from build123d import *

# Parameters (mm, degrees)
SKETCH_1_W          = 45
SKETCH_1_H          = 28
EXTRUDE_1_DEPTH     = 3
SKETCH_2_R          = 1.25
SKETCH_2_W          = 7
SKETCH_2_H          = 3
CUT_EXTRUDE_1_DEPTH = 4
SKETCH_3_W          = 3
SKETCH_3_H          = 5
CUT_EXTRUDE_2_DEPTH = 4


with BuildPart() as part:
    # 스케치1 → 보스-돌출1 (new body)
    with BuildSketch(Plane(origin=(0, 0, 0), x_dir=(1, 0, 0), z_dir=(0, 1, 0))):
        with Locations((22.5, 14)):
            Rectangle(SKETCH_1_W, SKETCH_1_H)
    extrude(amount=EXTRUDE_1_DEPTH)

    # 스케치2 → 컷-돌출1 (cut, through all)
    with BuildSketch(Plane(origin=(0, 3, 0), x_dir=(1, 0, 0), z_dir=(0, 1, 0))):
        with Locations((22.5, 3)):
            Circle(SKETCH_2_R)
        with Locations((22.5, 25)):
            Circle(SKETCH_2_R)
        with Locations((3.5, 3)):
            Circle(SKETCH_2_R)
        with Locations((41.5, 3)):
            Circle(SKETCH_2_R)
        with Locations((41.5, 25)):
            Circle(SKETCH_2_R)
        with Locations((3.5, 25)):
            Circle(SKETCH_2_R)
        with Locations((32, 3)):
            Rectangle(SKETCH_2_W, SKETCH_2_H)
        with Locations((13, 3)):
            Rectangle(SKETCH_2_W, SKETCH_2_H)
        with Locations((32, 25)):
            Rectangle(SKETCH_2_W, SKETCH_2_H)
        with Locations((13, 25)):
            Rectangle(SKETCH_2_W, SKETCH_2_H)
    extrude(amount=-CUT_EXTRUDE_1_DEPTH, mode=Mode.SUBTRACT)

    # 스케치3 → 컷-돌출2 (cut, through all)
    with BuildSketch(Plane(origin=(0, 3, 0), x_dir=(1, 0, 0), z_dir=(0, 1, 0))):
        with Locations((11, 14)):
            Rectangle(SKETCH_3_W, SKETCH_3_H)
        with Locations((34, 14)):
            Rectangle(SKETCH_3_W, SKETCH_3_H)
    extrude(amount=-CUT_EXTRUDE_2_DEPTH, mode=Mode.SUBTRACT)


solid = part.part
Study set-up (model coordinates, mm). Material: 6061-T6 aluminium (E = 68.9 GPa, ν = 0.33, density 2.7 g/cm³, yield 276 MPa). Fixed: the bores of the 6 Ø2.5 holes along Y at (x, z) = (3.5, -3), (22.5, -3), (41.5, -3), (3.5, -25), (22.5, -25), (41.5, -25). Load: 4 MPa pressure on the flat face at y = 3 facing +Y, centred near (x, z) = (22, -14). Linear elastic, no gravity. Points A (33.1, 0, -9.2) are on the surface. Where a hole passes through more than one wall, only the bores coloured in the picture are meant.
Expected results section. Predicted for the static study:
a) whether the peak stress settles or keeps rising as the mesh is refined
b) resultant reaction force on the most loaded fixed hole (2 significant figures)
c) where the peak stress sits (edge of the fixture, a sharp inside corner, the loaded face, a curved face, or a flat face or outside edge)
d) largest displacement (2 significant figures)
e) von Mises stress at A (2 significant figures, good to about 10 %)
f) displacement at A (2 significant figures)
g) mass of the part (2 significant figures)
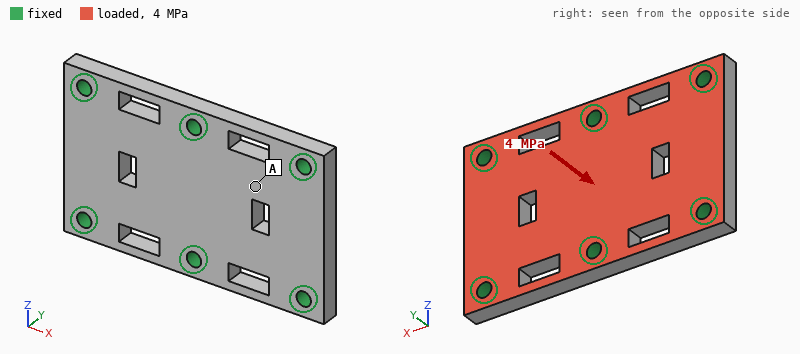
keeps rising
960 N
edge of the fixture
33 µm
41 MPa
26 µm
9.0 g
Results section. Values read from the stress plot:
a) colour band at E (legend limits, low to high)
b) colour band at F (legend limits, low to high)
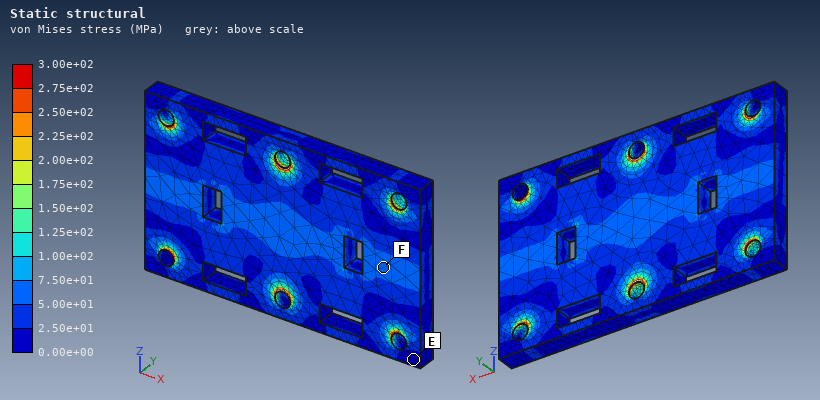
0.00e+00 to 2.50e+01 MPa
5.00e+01 to 7.50e+01 MPa
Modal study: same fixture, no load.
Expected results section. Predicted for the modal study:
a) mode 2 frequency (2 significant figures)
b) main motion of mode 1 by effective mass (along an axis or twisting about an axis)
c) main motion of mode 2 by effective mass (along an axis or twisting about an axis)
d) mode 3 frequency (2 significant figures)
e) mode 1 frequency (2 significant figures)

26 kHz
along Y
twisting about Z
35 kHz
24 kHz
